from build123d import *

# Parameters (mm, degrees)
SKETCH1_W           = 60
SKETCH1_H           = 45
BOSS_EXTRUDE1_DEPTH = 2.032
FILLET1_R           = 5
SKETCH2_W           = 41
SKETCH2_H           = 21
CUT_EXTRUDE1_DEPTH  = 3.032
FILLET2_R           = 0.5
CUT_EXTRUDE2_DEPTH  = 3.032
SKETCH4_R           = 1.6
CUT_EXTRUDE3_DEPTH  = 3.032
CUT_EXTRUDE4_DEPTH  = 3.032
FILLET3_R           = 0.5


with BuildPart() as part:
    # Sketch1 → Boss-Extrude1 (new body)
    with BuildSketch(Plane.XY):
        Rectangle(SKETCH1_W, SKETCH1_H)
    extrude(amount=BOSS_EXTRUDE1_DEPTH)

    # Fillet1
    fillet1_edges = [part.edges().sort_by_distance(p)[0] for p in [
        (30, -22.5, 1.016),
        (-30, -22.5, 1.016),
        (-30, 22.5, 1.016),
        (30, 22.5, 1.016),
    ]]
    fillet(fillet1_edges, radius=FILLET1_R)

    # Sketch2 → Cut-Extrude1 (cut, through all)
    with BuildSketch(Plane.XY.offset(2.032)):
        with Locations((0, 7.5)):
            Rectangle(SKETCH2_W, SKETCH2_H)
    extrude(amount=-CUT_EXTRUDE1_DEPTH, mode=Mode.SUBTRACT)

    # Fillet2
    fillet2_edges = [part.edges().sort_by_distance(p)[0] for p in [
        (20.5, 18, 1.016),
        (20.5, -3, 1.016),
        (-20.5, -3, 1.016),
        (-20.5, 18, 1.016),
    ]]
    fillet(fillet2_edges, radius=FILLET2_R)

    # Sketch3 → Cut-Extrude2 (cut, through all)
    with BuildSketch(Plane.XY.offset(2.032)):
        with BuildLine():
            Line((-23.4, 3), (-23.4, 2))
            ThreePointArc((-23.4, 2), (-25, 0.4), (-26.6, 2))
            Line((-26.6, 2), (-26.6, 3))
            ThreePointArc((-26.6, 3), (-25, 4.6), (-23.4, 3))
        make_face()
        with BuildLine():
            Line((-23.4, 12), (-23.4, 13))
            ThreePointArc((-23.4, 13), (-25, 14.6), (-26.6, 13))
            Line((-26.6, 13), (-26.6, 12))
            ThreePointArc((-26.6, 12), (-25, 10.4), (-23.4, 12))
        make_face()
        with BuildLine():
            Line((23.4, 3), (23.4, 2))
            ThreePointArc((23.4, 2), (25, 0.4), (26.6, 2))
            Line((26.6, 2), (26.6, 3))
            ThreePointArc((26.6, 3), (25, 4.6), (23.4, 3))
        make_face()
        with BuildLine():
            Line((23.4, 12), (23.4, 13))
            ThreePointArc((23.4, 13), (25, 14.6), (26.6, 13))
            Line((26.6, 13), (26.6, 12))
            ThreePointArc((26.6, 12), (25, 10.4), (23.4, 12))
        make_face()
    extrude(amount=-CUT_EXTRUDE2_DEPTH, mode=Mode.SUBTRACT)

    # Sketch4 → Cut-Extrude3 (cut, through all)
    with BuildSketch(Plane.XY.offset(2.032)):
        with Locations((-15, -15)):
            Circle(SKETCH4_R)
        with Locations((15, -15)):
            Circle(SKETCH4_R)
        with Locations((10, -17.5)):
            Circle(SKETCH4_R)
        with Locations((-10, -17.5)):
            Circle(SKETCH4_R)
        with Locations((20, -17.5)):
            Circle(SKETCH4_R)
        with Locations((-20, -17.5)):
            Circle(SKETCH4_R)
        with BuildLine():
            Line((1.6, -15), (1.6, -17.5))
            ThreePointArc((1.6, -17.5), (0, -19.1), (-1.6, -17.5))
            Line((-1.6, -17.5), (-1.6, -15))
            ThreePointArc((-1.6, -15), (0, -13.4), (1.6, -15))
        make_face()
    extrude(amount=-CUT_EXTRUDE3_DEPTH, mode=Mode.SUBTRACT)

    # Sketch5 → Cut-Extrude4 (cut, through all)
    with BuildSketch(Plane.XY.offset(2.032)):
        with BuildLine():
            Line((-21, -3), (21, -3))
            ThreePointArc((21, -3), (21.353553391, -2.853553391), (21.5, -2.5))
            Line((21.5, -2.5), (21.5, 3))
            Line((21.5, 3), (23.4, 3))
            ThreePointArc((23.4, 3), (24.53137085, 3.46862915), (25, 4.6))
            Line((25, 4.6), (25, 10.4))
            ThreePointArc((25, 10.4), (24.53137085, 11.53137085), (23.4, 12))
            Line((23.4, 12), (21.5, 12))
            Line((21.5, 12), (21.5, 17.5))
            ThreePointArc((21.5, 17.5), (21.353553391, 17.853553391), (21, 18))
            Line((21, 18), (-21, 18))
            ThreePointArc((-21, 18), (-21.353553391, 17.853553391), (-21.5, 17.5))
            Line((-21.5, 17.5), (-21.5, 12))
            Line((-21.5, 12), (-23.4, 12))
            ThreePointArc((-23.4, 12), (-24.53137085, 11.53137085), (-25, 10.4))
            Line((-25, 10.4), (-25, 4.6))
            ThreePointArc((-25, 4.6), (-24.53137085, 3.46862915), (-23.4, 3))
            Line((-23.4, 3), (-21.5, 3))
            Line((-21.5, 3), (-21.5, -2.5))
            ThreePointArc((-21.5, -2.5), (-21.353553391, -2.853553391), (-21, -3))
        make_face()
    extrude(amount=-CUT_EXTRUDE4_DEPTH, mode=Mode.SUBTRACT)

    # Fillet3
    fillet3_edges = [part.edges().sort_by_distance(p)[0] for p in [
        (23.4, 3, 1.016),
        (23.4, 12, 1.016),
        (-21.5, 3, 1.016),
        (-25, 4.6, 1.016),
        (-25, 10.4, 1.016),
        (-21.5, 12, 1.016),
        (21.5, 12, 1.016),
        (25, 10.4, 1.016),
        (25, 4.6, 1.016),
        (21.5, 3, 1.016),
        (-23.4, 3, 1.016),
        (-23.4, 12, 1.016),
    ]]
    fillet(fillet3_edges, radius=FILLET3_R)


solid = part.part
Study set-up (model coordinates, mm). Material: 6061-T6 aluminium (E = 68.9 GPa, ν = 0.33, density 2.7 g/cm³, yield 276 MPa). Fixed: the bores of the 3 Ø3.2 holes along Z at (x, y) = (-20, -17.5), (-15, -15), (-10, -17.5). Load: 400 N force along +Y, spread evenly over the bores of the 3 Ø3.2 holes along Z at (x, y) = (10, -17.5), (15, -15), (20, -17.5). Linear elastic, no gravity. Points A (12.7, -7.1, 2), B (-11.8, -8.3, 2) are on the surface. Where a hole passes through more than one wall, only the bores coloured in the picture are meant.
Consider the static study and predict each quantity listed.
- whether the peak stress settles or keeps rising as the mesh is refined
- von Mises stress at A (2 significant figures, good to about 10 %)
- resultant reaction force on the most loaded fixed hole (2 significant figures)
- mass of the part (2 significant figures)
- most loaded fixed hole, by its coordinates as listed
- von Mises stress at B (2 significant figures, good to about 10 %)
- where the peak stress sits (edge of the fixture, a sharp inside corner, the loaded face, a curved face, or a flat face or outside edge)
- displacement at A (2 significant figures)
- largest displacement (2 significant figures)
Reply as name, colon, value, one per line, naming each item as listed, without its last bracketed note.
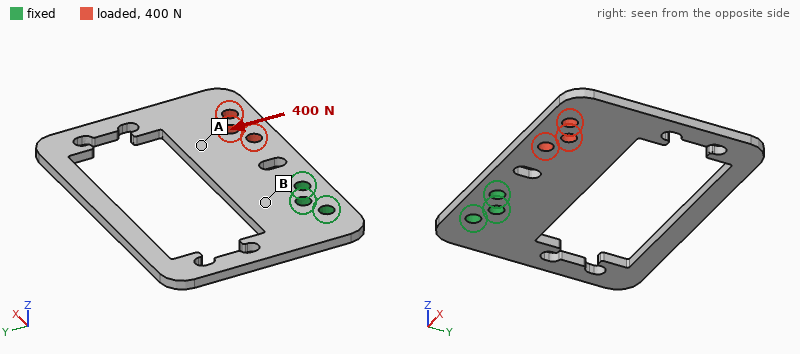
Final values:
whether the peak stress settles or keeps rising as the mesh is refined: keeps rising
von Mises stress at A: 13 MPa
resultant reaction force on the most loaded fixed hole: 1.1 kN
mass of the part: 8.8 g
most loaded fixed hole, by its coordinates as listed: (-10, -17.5)
von Mises stress at B: 38 MPa
where the peak stress sits: edge of the fixture
displacement at A: 0.063 mm
largest displacement: 0.12 mm
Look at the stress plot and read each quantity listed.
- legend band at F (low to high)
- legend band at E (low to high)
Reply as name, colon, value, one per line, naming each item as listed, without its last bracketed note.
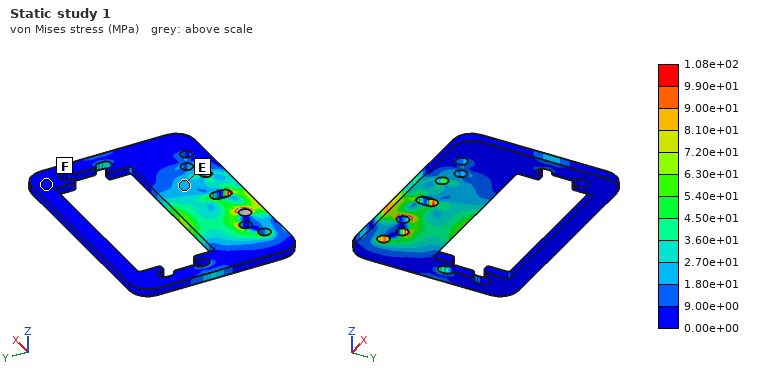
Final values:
legend band at F: 0.00e+00 to 9.00e+00 MPa
legend band at E: 1.80e+01 to 2.70e+01 MPa
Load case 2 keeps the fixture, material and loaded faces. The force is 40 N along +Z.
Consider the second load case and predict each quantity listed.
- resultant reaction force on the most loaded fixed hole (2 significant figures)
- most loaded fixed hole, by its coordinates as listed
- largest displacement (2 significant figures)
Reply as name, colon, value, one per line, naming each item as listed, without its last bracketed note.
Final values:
resultant reaction force on the most loaded fixed hole: 92 N
most loaded fixed hole, by its coordinates as listed: (-10, -17.5)
largest displacement: 0.46 mm
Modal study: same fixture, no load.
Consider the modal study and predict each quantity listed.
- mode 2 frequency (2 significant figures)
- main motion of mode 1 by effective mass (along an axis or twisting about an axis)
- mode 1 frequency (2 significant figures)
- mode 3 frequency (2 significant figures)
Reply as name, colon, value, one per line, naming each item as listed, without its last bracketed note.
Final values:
mode 2 frequency: 980 Hz
main motion of mode 1 by effective mass: along Z
mode 1 frequency: 590 Hz
mode 3 frequency: 1700 Hz
